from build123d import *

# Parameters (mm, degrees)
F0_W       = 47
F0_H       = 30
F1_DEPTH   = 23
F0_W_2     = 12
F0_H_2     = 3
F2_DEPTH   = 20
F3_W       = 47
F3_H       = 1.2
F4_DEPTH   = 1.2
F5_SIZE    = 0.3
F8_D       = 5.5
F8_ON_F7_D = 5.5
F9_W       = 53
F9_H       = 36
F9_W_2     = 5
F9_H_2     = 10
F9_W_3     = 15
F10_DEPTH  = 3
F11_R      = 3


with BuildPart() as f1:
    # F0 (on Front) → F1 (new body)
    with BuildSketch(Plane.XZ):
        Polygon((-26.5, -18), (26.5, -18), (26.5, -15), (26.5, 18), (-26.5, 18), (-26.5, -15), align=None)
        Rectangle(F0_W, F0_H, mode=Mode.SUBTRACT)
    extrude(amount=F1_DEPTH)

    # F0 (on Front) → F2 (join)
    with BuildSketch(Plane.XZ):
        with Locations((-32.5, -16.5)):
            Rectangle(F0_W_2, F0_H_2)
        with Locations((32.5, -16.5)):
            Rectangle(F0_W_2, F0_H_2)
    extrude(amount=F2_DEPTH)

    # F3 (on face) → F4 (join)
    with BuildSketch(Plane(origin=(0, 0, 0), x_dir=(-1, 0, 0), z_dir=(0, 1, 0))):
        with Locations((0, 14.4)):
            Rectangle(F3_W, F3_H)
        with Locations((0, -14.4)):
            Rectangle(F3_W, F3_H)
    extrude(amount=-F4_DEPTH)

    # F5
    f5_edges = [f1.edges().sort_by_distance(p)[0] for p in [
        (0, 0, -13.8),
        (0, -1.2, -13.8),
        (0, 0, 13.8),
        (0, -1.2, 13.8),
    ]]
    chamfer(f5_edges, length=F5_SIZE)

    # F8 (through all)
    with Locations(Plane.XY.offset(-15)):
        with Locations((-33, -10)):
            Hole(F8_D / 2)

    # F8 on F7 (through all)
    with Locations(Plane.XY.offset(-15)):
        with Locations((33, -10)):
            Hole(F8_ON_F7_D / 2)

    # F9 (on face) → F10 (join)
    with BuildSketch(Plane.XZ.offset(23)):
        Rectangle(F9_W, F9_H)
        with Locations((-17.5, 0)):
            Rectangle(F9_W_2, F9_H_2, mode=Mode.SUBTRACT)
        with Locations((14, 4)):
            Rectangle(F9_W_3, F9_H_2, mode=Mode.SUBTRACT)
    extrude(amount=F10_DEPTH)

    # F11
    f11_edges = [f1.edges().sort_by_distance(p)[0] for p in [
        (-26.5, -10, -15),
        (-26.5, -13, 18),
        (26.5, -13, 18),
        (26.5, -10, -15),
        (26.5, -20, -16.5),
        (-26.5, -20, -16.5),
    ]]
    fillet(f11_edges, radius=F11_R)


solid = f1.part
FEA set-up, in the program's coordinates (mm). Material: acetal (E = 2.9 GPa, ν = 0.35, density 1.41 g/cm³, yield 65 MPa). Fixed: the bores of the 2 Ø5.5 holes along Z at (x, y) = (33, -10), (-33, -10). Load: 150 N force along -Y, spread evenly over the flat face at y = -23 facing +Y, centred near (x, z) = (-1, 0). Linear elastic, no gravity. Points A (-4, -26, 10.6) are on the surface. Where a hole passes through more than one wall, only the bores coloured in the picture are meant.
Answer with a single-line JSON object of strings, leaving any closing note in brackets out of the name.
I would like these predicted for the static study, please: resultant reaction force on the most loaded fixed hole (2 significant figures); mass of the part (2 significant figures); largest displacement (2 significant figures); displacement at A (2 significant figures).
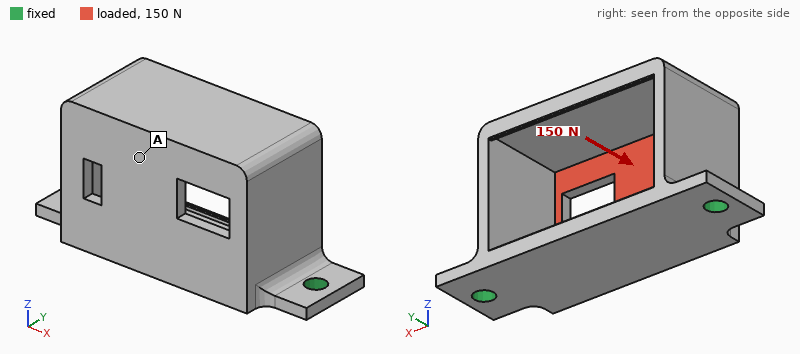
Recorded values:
{"resultant reaction force on the most loaded fixed hole": "79 N", "mass of the part": "25 g", "largest displacement": "0.87 mm", "displacement at A": "0.75 mm"}
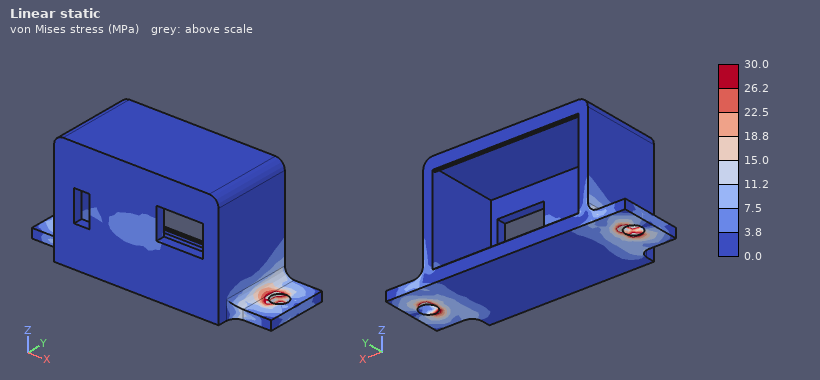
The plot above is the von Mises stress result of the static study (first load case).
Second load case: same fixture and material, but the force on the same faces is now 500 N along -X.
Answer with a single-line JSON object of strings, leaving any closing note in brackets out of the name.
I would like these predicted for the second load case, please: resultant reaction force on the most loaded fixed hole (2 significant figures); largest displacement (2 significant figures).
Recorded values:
{"resultant reaction force on the most loaded fixed hole": "300 N", "largest displacement": "0.90 mm"}
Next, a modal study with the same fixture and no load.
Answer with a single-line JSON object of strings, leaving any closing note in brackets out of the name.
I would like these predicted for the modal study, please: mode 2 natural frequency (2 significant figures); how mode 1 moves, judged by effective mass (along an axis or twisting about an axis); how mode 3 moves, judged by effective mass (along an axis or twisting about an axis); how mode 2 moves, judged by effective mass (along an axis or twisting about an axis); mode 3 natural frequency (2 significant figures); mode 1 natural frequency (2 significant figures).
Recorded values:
{"mode 2 natural frequency": "710 Hz", "how mode 1 moves, judged by effective mass": "along Y", "how mode 3 moves, judged by effective mass": "along Z", "how mode 2 moves, judged by effective mass": "along X", "mode 3 natural frequency": "1600 Hz", "mode 1 natural frequency": "470 Hz"}
